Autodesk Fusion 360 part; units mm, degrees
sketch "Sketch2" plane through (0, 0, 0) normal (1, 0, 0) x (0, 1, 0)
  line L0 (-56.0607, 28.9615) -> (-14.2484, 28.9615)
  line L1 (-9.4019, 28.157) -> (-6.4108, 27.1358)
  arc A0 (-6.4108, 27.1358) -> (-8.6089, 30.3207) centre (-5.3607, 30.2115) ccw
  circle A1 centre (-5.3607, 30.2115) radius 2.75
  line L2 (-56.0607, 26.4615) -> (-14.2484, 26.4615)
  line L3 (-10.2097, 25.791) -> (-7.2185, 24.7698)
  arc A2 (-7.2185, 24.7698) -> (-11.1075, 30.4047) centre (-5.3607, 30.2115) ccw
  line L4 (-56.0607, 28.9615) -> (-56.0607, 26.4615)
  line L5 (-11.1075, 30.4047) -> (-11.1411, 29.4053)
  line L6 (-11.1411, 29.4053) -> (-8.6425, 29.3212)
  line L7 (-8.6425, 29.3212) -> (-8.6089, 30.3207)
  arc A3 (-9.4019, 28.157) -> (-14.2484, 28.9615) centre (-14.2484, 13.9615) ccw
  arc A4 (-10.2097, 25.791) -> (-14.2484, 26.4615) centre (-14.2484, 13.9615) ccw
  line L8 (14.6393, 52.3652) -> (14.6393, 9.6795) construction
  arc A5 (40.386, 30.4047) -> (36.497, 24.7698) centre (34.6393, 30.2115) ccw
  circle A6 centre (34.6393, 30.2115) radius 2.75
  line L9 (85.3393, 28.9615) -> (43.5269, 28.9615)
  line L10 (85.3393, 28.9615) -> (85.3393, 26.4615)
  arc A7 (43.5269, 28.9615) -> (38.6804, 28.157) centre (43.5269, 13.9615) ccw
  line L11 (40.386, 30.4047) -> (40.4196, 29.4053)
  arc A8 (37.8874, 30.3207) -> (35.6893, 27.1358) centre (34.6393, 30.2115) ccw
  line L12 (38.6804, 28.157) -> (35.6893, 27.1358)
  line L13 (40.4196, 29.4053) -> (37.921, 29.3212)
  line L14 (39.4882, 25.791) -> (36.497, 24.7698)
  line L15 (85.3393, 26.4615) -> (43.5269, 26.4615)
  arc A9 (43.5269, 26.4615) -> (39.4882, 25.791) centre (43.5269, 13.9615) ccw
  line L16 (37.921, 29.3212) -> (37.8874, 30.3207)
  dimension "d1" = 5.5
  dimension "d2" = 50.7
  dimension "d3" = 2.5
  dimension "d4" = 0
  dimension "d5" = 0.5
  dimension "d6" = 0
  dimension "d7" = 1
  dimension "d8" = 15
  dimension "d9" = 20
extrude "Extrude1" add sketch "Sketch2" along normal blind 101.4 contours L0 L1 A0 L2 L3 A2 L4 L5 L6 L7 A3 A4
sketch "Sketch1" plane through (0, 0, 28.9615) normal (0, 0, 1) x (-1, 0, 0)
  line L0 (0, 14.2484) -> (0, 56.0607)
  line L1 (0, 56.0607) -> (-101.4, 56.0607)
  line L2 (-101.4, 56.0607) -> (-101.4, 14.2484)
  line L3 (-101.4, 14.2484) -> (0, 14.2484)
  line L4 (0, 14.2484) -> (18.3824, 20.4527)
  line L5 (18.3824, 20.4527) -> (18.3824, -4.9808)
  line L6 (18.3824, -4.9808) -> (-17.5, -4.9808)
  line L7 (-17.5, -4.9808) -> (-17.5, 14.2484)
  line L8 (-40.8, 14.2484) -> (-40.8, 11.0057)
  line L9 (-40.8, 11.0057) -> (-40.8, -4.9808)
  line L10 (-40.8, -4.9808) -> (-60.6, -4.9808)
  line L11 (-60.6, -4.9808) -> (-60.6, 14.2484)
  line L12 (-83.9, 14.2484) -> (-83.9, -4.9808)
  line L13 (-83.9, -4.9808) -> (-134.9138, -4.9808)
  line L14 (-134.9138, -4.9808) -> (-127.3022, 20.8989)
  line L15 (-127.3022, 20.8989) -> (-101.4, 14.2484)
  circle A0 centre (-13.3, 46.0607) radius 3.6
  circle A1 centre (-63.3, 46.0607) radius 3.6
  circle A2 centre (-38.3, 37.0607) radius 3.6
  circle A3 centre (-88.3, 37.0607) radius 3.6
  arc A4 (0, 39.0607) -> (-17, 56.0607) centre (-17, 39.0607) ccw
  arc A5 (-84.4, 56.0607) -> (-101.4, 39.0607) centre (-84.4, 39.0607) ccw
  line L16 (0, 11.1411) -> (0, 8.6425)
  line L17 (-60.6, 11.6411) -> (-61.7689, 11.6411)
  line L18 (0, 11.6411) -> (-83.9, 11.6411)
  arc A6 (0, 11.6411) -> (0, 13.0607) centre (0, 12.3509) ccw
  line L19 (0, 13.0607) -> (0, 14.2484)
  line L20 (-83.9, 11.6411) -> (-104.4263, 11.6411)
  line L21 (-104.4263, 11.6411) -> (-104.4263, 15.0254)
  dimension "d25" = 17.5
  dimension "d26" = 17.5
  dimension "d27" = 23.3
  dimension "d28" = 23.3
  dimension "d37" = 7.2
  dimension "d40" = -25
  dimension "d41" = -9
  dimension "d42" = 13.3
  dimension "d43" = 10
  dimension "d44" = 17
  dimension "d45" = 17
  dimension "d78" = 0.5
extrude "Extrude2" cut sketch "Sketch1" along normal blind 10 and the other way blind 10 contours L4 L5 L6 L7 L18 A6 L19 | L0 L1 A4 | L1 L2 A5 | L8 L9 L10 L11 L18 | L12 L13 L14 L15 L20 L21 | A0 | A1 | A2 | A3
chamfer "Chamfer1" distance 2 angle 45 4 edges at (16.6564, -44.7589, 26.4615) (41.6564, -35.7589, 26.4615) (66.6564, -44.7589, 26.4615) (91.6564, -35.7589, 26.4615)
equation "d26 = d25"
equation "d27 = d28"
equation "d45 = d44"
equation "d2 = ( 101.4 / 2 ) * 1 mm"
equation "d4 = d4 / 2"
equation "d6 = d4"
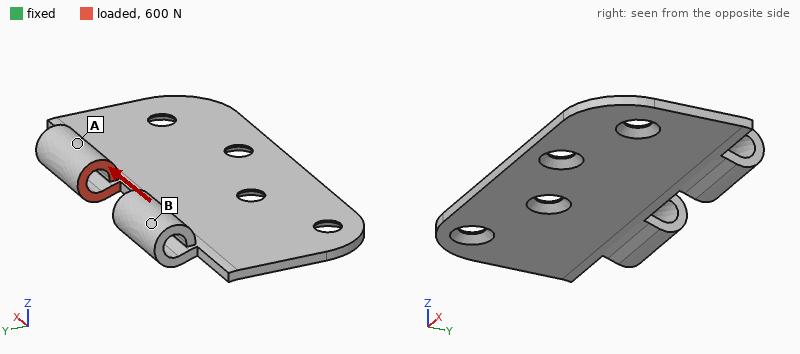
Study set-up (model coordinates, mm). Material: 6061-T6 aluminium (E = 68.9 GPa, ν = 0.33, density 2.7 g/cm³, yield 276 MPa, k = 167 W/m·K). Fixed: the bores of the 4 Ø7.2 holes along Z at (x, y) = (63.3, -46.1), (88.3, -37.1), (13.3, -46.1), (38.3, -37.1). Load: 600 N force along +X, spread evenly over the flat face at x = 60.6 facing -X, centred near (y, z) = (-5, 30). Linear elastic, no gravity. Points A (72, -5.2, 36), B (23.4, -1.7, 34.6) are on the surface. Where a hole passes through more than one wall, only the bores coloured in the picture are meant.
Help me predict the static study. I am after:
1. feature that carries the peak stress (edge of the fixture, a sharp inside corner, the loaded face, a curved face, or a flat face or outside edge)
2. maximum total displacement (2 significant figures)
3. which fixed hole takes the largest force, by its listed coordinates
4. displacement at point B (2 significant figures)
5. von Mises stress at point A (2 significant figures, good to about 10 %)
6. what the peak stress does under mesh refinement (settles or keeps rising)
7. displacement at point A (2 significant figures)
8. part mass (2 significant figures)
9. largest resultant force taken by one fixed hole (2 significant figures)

edge of the fixture
0.21 mm
(88.3, -37.1)
0.048 mm
19 MPa
keeps rising
0.14 mm
37 g
420 N
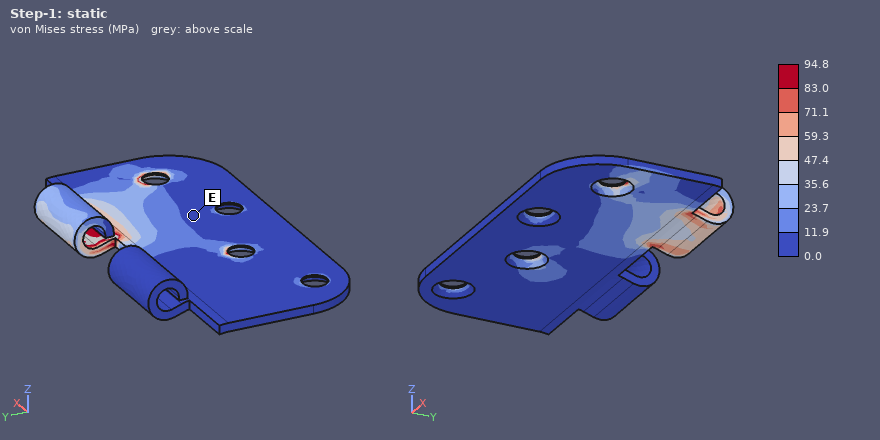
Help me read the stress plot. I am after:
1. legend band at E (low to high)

0.0 to 11.9 MPa
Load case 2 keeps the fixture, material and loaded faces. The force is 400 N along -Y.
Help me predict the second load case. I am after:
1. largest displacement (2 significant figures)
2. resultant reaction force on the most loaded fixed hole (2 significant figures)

0.22 mm
160 N
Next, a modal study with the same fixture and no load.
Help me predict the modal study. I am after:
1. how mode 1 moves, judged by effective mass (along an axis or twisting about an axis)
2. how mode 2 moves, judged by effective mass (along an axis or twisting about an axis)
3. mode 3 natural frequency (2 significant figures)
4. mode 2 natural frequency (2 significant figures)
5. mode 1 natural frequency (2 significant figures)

along Z
twisting about Y
2800 Hz
1400 Hz
1000 Hz
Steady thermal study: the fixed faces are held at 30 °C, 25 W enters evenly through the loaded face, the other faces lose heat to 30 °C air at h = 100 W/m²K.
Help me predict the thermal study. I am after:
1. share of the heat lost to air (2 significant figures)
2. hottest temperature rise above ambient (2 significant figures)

44 %
68 K
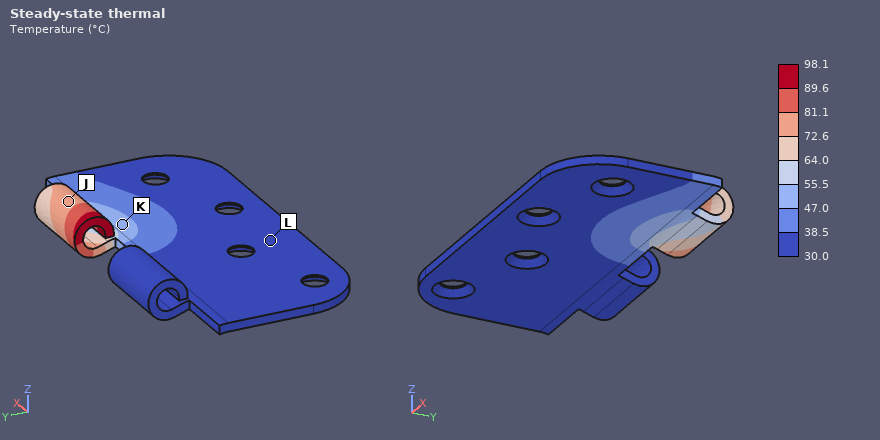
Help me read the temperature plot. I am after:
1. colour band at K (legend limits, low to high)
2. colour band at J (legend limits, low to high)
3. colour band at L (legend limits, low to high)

47.0 to 55.5 °C
72.6 to 81.1 °C
30.0 to 38.5 °C
